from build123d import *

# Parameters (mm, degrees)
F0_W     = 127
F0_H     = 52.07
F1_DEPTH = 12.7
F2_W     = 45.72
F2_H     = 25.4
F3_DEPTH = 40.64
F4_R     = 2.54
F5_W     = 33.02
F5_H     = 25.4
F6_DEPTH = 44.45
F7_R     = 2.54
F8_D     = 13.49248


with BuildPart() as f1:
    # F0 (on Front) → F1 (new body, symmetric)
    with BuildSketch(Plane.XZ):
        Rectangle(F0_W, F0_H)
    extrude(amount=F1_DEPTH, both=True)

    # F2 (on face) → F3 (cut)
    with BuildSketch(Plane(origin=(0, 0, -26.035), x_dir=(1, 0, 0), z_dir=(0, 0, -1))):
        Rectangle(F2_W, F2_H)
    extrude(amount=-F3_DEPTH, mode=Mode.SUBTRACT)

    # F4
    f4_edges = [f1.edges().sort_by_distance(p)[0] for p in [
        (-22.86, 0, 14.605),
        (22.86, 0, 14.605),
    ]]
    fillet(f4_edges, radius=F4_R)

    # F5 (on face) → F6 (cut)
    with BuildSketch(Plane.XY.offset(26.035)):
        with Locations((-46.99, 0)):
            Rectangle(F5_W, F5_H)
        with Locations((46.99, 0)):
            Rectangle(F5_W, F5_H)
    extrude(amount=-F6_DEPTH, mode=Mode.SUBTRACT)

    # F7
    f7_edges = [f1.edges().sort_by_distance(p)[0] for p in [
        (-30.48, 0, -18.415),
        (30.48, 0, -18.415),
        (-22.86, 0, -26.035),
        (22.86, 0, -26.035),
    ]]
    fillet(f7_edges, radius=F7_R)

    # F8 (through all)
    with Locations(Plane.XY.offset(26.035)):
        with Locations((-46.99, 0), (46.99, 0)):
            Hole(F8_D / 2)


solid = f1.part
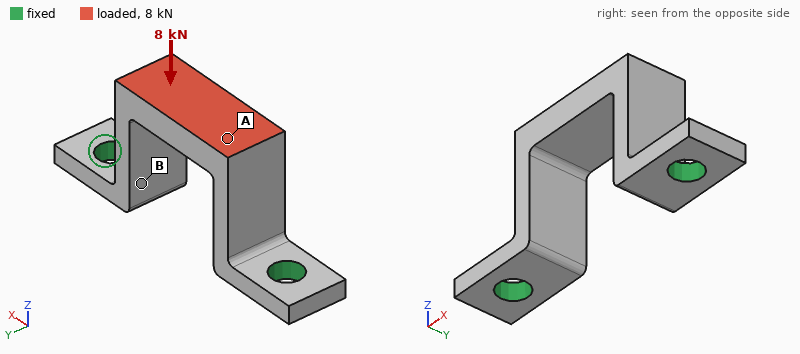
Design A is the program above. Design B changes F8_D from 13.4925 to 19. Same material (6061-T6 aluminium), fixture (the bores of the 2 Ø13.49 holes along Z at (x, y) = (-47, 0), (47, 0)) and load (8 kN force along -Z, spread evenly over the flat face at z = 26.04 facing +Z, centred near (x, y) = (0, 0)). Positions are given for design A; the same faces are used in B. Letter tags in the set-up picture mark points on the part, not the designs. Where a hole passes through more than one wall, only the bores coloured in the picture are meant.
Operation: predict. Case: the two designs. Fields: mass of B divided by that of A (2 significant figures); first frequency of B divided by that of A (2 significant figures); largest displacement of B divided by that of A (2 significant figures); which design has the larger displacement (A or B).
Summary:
0.95
1.2
0.83
A
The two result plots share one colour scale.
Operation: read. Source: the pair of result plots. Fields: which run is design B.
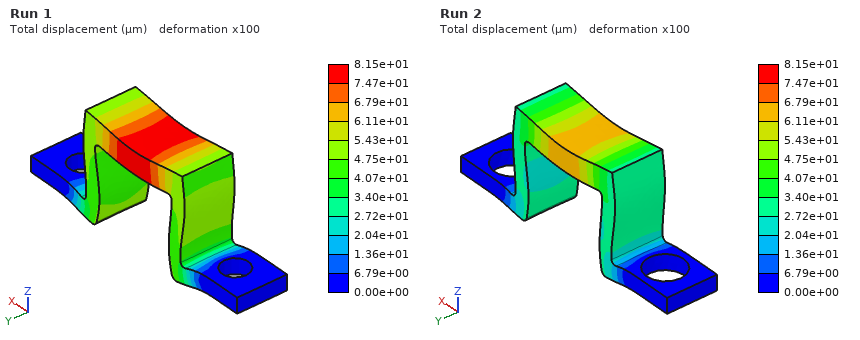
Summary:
Run 2
